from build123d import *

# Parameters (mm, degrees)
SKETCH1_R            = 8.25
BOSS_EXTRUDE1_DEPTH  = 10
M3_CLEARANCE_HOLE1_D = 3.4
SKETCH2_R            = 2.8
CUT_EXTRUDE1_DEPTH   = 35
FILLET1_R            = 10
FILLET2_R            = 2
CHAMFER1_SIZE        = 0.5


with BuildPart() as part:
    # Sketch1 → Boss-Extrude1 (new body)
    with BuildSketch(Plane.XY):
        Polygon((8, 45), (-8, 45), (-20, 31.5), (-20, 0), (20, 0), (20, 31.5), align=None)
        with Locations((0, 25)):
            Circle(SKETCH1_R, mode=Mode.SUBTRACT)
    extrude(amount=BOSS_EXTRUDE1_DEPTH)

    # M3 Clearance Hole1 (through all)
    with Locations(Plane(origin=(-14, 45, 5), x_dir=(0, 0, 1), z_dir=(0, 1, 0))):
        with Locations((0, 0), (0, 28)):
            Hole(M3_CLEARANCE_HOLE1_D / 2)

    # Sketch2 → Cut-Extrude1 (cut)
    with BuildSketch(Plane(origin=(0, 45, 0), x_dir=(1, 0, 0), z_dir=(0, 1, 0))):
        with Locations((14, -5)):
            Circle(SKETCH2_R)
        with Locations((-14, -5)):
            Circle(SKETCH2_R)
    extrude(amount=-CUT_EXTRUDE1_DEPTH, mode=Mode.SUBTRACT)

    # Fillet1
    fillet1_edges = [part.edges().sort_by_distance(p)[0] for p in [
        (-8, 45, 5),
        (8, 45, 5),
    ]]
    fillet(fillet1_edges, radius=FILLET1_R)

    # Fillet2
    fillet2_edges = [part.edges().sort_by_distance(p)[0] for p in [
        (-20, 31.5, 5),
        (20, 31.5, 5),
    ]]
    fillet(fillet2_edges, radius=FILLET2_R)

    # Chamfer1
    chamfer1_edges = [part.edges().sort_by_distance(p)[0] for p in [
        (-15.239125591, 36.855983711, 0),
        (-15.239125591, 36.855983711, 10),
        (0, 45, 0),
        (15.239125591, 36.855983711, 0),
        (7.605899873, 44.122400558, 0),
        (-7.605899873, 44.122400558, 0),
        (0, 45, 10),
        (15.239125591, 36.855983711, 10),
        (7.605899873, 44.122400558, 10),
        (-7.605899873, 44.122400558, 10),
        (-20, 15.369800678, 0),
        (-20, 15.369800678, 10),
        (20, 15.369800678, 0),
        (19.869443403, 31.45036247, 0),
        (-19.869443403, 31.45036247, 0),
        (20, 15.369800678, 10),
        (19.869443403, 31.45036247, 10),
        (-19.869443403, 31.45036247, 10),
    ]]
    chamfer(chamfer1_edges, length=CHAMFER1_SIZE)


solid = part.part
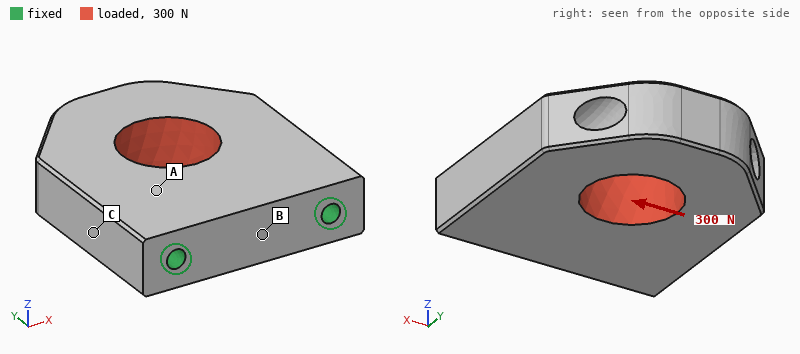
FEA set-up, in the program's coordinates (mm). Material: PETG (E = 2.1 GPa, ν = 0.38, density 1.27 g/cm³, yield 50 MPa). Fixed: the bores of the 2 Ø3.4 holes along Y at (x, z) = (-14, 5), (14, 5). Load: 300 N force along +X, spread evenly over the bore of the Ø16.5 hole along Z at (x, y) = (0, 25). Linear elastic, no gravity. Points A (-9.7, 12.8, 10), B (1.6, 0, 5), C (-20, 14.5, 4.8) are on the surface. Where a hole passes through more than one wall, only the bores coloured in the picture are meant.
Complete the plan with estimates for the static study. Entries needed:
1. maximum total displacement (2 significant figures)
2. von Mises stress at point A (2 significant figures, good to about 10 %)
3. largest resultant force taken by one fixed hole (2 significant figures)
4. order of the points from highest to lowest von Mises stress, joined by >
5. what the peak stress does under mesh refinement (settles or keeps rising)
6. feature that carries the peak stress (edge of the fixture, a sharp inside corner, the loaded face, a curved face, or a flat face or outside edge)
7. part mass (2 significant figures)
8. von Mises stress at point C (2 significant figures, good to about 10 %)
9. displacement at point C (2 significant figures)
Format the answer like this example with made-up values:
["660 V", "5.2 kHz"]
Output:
["84 µm", "1.3 MPa", "230 N", "C > A > B", "keeps rising", "edge of the fixture", "16 g", "2.3 MPa", "27 µm"]
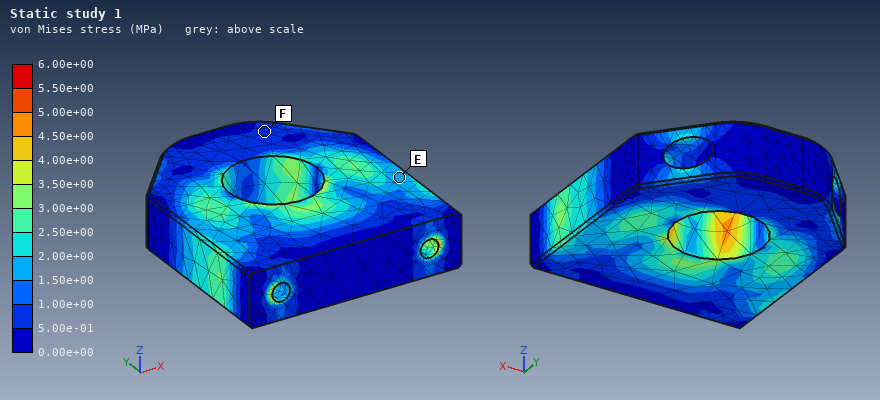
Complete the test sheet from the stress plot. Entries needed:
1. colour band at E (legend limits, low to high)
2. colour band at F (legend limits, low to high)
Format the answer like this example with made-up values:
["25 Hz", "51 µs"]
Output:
["1.50e+00 to 2.00e+00 MPa", "5.00e-01 to 1.00e+00 MPa"]
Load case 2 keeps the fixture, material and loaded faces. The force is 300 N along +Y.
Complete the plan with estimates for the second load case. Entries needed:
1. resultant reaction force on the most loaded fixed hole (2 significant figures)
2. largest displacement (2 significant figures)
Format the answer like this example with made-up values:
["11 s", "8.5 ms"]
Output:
["150 N", "24 µm"]
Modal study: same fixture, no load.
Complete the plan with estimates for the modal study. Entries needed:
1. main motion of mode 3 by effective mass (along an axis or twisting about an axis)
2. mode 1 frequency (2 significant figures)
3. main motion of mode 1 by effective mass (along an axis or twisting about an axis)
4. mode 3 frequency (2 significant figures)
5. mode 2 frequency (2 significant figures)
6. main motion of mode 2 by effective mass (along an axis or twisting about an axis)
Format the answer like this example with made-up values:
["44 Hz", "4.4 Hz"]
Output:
["twisting about Y", "1200 Hz", "along Z", "3300 Hz", "3000 Hz", "along X"]
